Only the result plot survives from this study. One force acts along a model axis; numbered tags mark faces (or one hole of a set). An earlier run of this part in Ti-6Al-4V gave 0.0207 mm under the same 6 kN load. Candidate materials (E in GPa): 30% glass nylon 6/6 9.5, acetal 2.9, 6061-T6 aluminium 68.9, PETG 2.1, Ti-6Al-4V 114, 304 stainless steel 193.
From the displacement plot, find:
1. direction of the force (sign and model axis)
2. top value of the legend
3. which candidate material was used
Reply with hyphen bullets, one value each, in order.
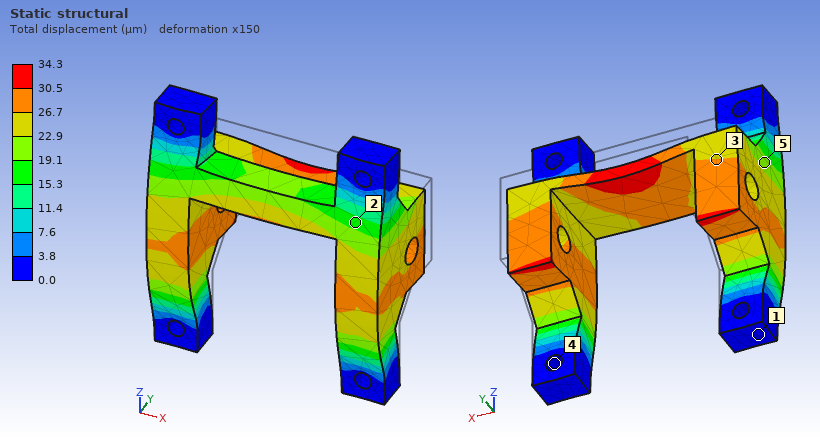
- -Y
- 34.3 µm
- 6061-T6 aluminium
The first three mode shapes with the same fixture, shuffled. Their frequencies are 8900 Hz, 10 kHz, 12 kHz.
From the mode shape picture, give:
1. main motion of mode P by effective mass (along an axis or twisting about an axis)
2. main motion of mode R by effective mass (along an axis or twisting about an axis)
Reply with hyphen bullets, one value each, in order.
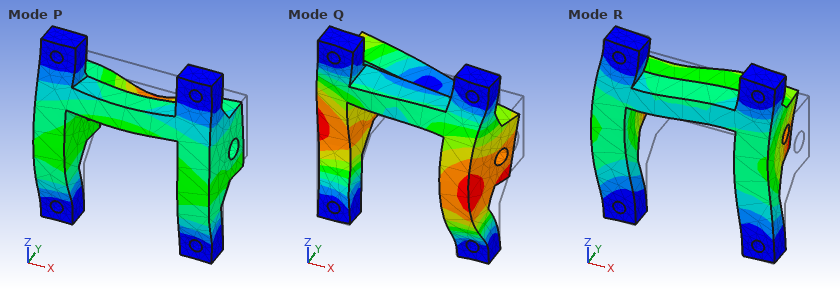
- along Y
- along X
